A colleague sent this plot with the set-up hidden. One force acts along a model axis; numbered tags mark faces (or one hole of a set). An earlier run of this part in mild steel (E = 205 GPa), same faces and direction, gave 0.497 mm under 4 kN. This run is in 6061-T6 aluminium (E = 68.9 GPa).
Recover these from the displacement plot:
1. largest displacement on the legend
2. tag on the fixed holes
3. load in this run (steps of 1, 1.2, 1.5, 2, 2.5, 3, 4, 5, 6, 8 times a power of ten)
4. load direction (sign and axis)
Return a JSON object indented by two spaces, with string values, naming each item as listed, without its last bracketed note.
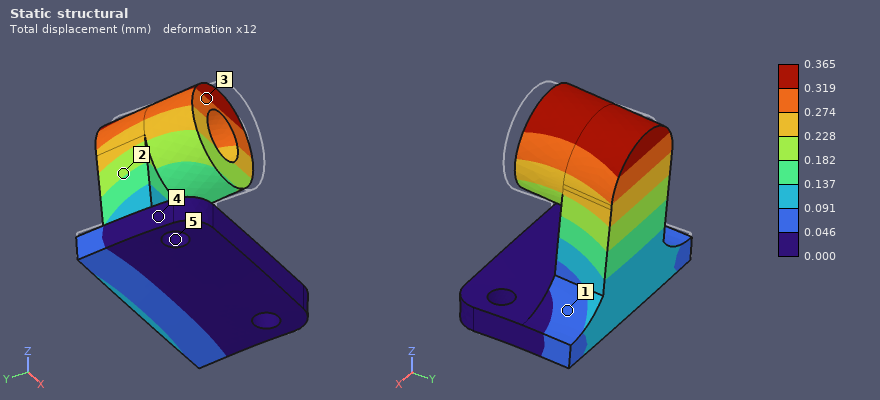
{
  "largest displacement on the legend": "0.365 mm",
  "tag on the fixed holes": "5",
  "load in this run": "1 kN",
  "load direction": "+Y"
}
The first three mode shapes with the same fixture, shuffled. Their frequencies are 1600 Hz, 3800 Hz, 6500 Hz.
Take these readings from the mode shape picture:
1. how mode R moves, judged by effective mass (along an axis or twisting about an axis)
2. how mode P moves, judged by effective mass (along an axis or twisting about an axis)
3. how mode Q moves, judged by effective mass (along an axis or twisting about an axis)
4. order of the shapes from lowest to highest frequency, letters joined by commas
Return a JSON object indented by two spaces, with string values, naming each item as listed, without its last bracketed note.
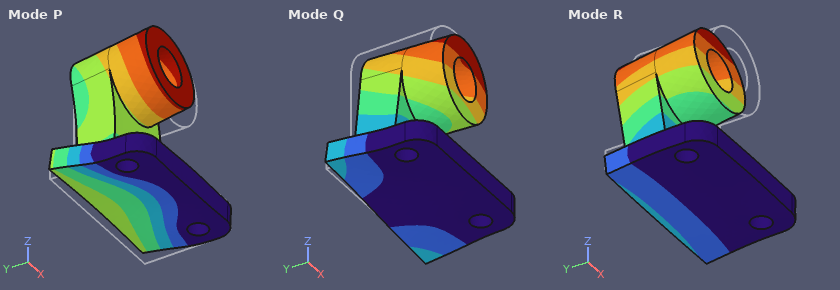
{
  "how mode R moves, judged by effective mass": "along Y",
  "how mode P moves, judged by effective mass": "along Z",
  "how mode Q moves, judged by effective mass": "along X",
  "order of the shapes from lowest to highest frequency, letters joined by commas": "R, Q, P"
}
